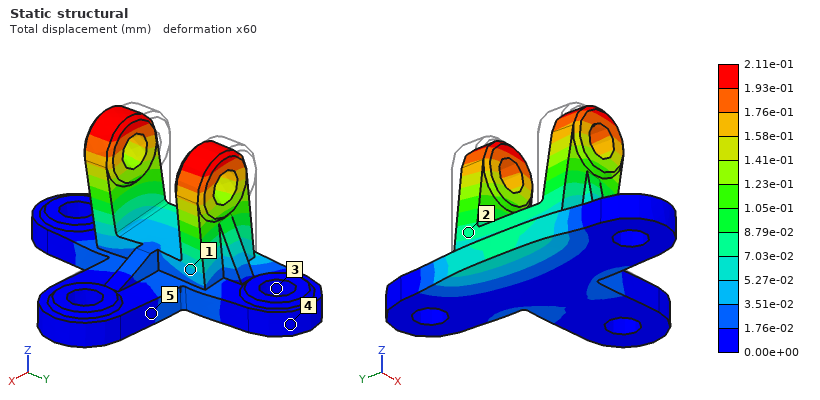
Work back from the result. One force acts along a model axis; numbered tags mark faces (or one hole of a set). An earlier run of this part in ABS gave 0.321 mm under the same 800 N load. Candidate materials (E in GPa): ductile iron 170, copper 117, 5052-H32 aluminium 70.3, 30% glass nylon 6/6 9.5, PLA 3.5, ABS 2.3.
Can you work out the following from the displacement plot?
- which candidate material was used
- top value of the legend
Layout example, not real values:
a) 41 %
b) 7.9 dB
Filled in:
a) PLA
b) 2.11e-01 mm
